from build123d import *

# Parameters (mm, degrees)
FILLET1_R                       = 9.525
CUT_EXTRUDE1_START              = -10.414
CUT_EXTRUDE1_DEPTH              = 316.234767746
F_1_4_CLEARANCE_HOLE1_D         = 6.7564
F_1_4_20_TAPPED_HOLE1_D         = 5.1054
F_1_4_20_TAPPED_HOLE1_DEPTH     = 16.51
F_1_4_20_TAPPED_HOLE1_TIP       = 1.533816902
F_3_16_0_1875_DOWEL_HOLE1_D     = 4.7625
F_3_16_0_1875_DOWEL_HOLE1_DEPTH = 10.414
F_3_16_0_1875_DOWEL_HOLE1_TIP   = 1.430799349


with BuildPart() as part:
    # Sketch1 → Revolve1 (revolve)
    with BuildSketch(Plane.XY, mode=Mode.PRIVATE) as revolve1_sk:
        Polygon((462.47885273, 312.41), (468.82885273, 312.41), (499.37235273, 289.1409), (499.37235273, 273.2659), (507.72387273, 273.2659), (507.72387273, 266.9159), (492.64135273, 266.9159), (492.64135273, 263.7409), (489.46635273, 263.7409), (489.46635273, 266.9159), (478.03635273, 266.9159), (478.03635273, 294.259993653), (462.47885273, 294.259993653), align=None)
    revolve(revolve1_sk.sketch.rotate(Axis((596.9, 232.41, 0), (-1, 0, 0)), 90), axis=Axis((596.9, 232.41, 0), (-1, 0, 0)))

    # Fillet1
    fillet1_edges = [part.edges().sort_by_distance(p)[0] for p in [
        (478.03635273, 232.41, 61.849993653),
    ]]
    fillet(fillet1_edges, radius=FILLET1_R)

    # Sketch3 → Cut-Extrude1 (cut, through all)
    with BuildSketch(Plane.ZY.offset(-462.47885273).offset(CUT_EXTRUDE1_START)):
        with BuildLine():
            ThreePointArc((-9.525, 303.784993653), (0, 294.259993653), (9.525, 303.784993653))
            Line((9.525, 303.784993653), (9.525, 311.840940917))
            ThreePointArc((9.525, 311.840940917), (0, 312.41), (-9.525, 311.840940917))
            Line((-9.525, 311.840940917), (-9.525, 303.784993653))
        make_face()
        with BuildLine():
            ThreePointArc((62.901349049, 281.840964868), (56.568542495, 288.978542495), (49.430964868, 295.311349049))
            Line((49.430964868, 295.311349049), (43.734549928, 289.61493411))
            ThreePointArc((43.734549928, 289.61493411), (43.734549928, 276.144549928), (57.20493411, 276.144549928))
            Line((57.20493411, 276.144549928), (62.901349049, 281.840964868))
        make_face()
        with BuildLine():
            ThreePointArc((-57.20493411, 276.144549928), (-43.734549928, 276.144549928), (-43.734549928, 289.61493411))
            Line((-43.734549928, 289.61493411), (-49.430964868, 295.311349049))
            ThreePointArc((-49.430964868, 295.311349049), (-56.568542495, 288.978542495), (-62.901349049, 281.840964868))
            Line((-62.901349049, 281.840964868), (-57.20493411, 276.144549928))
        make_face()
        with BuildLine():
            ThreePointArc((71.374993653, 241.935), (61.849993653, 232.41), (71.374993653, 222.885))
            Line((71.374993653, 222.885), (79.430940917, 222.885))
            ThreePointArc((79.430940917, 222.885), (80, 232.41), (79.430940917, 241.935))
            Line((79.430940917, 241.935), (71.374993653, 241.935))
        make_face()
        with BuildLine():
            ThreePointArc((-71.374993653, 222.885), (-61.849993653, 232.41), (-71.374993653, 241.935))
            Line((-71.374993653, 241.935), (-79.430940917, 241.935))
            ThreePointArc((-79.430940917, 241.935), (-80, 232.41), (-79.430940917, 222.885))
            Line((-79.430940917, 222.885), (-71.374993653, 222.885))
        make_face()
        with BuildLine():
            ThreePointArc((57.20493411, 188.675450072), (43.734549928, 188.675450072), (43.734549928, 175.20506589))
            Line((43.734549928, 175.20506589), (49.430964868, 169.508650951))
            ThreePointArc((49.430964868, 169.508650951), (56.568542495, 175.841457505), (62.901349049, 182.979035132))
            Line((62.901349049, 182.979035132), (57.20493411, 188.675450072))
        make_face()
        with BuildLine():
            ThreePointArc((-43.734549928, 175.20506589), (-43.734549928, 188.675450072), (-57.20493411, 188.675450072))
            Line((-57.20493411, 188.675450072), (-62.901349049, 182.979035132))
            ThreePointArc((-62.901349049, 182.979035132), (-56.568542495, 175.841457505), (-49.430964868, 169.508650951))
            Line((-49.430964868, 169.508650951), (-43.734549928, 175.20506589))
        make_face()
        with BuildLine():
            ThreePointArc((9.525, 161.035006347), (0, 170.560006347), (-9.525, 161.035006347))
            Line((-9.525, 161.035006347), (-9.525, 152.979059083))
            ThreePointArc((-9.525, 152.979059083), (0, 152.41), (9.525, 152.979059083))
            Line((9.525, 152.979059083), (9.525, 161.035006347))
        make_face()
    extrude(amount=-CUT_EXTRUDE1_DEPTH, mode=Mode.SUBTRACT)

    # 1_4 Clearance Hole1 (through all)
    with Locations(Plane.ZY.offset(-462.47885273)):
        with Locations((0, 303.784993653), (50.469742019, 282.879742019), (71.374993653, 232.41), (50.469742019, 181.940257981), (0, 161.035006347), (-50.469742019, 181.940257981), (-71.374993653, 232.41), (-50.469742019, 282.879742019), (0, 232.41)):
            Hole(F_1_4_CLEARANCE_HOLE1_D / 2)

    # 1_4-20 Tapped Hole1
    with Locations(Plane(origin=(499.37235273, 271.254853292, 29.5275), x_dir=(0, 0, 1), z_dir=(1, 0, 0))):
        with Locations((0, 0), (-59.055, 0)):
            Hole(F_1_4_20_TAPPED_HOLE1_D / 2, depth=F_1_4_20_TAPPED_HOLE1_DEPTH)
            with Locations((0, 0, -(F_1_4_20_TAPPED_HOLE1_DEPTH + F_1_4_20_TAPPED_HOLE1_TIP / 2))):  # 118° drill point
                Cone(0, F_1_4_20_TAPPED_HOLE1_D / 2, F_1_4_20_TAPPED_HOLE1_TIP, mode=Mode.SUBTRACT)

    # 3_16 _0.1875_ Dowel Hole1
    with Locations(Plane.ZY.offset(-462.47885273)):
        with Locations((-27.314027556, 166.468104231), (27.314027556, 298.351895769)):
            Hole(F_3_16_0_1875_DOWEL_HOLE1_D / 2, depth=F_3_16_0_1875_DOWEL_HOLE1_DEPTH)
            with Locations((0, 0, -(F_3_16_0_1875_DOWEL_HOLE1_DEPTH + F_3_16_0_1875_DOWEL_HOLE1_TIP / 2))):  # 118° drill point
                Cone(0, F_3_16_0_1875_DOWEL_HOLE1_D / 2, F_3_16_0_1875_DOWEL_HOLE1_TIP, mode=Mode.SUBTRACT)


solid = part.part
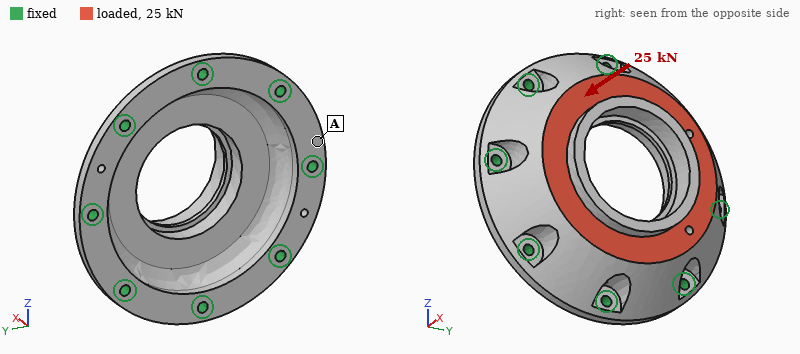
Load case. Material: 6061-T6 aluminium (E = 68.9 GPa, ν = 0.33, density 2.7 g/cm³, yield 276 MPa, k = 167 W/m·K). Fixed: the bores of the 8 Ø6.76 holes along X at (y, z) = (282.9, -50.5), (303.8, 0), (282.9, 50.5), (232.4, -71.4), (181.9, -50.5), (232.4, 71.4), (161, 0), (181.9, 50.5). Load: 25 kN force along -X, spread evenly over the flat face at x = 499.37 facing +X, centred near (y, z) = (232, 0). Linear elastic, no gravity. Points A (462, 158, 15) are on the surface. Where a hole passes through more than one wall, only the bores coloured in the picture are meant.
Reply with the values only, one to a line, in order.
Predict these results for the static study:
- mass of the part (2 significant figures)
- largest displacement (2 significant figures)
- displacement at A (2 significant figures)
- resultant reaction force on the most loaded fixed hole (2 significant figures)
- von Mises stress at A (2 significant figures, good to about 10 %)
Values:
850 g
19 µm
4.7 µm
3.8 kN
7.4 MPa
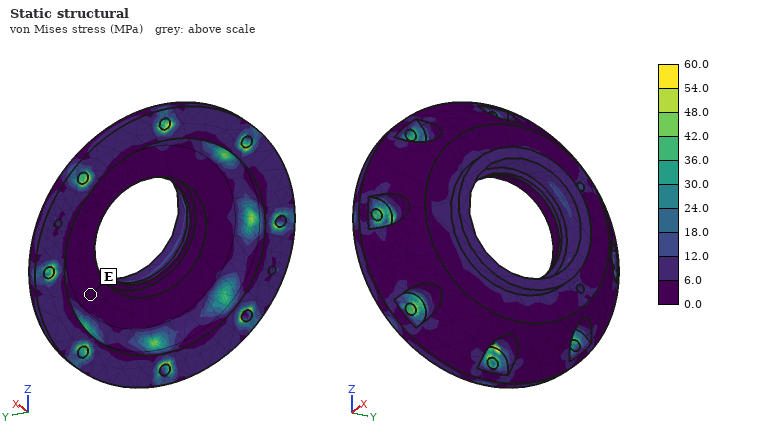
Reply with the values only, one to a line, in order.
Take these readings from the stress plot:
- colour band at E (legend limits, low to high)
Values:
0.0 to 6.0 MPa
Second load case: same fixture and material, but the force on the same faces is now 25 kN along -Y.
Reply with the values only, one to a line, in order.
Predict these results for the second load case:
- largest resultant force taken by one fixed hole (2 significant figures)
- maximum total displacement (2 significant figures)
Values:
3.9 kN
21 µm
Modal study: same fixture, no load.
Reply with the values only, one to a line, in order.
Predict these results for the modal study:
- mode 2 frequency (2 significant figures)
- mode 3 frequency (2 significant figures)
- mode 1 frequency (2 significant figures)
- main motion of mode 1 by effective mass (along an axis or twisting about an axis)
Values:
9200 Hz
9200 Hz
8600 Hz
along X
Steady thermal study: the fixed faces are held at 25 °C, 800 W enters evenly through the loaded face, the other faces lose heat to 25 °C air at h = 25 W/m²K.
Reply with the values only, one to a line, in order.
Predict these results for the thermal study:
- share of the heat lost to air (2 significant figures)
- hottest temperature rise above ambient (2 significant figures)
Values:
4.9 %
50 K
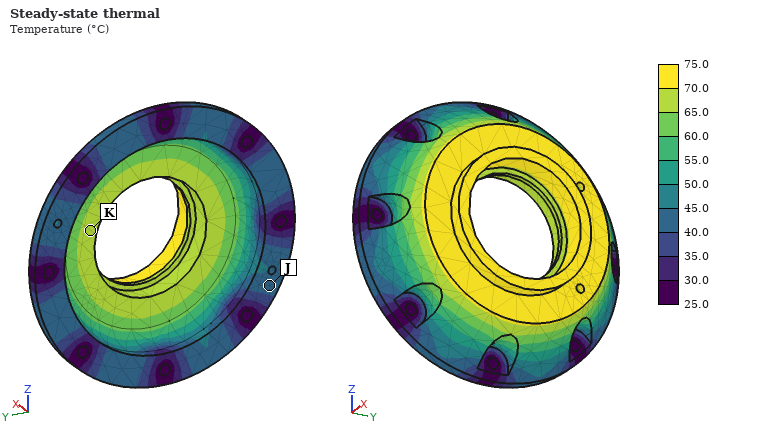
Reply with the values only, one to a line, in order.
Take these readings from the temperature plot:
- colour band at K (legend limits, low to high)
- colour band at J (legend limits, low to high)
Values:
65.0 to 70.0 °C
40.0 to 45.0 °C
